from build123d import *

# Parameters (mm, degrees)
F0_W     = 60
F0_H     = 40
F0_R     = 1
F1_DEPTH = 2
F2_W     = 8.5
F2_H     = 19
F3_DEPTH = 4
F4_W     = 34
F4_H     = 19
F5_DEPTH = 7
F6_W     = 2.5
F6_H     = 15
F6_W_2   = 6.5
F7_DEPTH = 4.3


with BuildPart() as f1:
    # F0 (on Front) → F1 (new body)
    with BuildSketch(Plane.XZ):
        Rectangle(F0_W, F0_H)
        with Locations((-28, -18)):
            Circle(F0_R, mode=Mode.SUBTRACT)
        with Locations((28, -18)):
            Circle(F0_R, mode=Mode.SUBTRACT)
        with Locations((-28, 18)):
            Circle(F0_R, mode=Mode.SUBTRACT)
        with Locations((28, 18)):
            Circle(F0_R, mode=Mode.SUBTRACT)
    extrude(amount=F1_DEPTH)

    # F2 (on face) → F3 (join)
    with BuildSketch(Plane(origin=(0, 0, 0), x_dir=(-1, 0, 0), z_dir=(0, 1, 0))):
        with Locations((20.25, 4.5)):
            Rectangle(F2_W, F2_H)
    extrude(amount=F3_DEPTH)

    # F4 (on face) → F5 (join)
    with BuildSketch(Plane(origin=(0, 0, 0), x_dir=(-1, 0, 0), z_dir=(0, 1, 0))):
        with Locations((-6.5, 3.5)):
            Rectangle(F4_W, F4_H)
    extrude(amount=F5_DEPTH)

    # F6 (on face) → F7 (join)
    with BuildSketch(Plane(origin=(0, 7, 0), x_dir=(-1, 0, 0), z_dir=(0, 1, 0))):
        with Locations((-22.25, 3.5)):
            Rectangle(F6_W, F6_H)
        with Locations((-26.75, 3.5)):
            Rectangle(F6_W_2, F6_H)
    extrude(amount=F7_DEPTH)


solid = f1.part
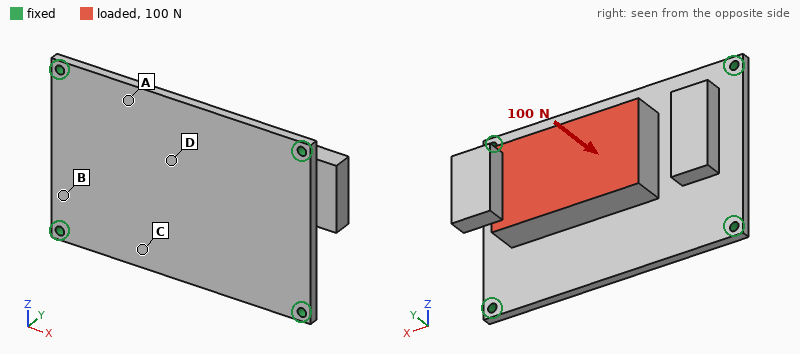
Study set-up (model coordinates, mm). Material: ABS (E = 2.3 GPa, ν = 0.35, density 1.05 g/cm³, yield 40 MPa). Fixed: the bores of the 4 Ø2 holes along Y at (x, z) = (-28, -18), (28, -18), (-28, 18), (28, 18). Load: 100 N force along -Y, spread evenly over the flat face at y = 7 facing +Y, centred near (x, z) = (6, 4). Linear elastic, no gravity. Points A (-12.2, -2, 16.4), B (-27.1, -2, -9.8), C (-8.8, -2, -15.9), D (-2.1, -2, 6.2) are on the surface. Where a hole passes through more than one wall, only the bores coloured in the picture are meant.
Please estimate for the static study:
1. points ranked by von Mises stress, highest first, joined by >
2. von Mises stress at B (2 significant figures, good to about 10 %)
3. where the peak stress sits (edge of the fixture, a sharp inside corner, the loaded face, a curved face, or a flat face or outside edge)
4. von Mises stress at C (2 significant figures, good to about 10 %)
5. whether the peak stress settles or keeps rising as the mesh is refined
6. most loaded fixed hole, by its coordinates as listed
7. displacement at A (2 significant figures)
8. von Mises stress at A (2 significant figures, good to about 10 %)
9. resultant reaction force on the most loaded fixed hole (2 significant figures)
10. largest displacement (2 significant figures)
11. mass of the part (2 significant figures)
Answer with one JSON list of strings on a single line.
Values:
["A > C > B > D", "5.2 MPa", "edge of the fixture", "7.8 MPa", "keeps rising", "(28, 18)", "0.50 mm", "11 MPa", "44 N", "0.66 mm", "11 g"]
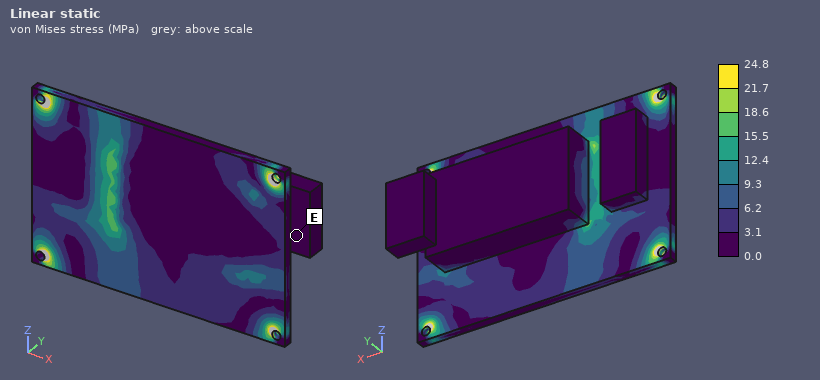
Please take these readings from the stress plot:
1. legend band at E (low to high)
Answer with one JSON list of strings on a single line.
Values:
["0.0 to 3.1 MPa"]
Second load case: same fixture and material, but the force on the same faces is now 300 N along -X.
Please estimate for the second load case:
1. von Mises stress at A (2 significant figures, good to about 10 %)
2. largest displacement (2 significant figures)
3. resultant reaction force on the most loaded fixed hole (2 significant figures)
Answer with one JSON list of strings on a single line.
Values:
["14 MPa", "0.66 mm", "110 N"]
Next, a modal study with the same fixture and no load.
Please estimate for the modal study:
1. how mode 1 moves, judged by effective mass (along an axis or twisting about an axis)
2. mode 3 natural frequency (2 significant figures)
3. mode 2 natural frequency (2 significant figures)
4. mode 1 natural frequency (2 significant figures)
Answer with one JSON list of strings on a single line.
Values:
["along Y", "1800 Hz", "1400 Hz", "750 Hz"]
